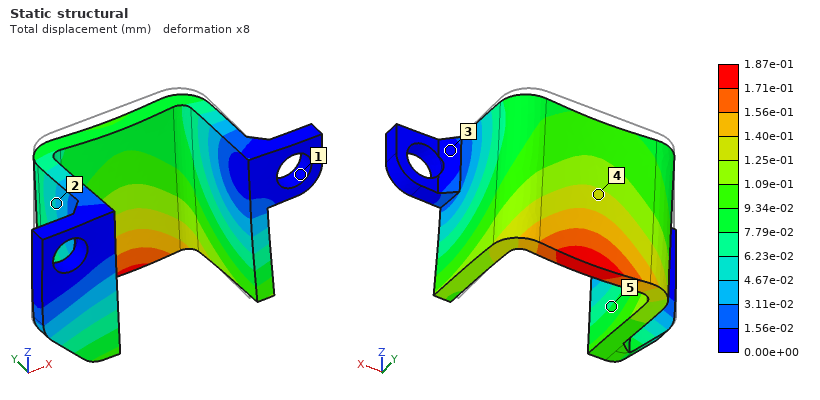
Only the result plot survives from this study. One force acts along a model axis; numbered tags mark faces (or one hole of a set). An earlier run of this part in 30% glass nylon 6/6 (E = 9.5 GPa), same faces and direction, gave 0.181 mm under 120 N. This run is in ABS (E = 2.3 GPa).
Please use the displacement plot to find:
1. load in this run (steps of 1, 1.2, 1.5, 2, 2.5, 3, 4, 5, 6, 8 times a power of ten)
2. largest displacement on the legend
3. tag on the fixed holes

30 N
1.87e-01 mm
1
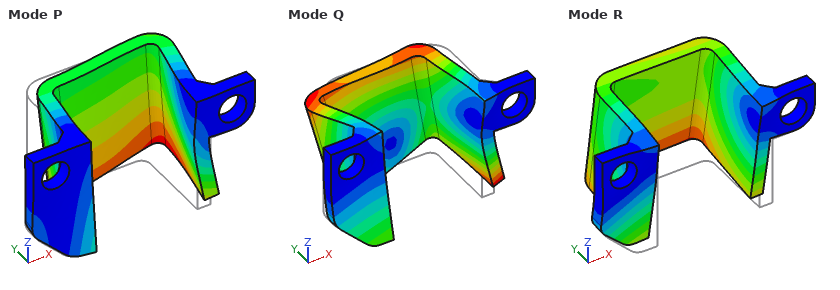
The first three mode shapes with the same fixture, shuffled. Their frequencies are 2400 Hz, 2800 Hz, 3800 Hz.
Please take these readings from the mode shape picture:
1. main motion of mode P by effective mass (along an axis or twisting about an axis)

along X
